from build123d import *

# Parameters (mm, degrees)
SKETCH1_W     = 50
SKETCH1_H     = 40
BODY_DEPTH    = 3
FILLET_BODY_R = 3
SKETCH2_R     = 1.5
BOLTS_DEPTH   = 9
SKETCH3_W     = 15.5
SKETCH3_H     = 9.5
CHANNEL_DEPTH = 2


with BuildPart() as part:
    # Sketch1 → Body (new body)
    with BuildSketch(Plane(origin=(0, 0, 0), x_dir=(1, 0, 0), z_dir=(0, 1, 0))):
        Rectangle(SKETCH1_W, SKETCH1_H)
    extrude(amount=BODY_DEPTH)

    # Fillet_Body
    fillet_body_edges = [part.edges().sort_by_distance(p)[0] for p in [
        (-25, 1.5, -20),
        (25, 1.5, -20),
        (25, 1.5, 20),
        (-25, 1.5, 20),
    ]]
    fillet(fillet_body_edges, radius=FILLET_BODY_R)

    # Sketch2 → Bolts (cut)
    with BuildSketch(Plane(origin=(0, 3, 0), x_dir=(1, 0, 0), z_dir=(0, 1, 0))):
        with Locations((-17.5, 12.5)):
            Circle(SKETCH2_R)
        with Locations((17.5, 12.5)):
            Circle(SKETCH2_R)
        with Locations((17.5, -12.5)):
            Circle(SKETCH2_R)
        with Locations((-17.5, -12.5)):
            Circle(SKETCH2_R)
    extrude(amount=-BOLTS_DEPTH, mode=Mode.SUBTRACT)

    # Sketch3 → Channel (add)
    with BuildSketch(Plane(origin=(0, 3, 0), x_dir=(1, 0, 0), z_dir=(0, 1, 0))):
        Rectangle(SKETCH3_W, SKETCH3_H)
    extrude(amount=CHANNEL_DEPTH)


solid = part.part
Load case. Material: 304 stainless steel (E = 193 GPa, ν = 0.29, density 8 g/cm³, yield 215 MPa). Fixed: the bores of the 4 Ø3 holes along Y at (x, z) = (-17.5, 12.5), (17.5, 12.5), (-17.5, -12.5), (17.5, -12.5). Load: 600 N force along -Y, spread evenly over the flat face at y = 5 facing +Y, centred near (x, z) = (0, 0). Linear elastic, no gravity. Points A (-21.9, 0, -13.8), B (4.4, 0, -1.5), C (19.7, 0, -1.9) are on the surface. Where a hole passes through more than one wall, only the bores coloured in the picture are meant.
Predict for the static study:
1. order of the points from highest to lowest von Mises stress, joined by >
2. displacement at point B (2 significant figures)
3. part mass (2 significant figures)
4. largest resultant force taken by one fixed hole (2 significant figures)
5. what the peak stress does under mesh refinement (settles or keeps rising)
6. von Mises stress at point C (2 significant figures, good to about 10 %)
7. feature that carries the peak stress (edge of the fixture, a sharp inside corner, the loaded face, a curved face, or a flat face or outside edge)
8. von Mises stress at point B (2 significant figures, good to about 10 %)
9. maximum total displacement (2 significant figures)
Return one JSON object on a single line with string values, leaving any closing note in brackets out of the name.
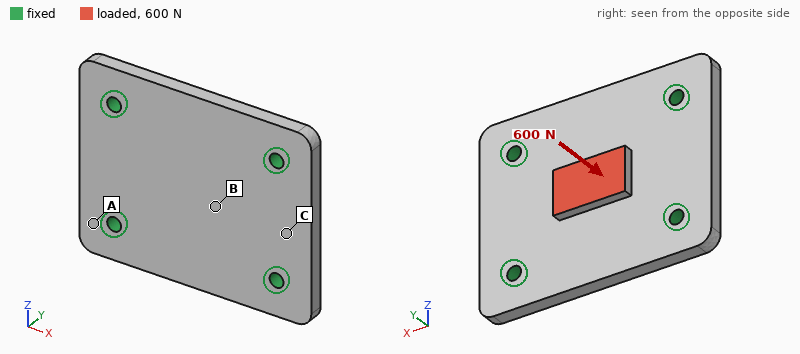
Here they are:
{"order of the points from highest to lowest von Mises stress, joined by >": "B > C > A", "displacement at point B": "8.4 µm", "part mass": "49 g", "largest resultant force taken by one fixed hole": "160 N", "what the peak stress does under mesh refinement": "keeps rising", "von Mises stress at point C": "12 MPa", "feature that carries the peak stress": "edge of the fixture", "von Mises stress at point B": "21 MPa", "maximum total displacement": "8.9 µm"}
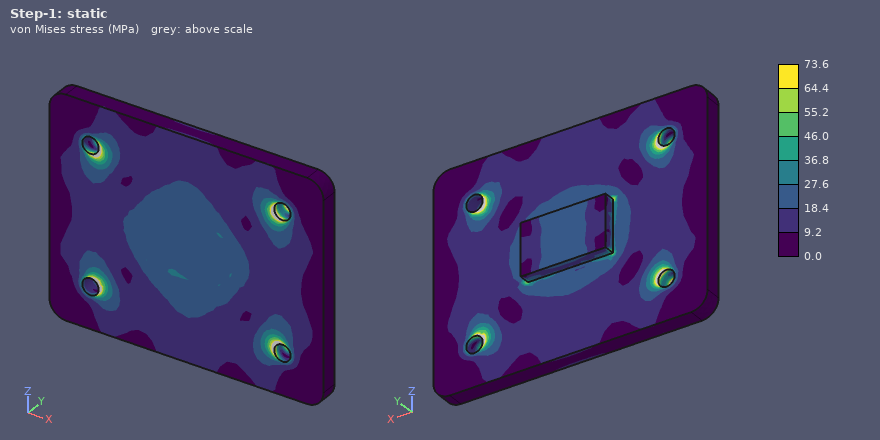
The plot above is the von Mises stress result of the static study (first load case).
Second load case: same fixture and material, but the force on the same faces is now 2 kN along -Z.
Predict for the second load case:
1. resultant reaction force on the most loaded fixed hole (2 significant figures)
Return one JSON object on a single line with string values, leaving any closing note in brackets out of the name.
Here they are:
{"resultant reaction force on the most loaded fixed hole": "580 N"}
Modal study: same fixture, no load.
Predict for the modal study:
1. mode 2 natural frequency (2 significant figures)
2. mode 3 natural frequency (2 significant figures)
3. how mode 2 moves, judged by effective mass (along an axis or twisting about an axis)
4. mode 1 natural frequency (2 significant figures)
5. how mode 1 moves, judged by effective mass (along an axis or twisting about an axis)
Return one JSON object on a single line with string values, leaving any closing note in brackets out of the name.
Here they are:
{"mode 2 natural frequency": "13 kHz", "mode 3 natural frequency": "17 kHz", "how mode 2 moves, judged by effective mass": "twisting about X", "mode 1 natural frequency": "11 kHz", "how mode 1 moves, judged by effective mass": "along Y"}
